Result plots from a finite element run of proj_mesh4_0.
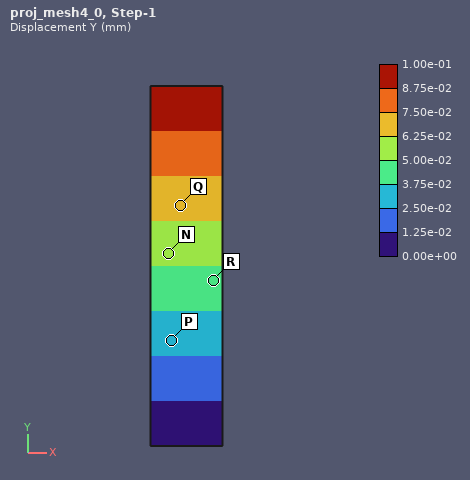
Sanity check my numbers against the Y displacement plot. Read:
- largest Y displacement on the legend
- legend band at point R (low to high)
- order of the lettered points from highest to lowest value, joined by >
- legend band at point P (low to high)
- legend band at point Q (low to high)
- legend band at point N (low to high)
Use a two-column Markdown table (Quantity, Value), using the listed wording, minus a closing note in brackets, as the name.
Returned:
| Quantity | Value |
|---|---|
| largest Y displacement on the legend | 1.00e-01 mm |
| legend band at point R | 3.75e-02 to 5.00e-02 mm |
| order of the lettered points from highest to lowest value, joined by > | Q > N > R > P |
| legend band at point P | 2.50e-02 to 3.75e-02 mm |
| legend band at point Q | 6.25e-02 to 7.50e-02 mm |
| legend band at point N | 5.00e-02 to 6.25e-02 mm |
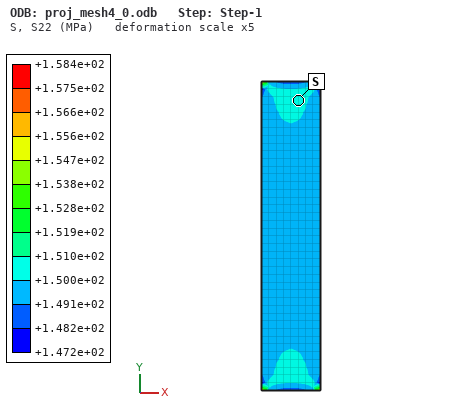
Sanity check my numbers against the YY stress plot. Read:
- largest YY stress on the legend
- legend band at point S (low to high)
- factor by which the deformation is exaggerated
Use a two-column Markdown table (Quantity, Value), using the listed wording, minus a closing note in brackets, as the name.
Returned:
| Quantity | Value |
|---|---|
| largest YY stress on the legend | +1.584e+02 MPa |
| legend band at point S | +1.500e+02 to +1.510e+02 MPa |
| factor by which the deformation is exaggerated | 5 |
